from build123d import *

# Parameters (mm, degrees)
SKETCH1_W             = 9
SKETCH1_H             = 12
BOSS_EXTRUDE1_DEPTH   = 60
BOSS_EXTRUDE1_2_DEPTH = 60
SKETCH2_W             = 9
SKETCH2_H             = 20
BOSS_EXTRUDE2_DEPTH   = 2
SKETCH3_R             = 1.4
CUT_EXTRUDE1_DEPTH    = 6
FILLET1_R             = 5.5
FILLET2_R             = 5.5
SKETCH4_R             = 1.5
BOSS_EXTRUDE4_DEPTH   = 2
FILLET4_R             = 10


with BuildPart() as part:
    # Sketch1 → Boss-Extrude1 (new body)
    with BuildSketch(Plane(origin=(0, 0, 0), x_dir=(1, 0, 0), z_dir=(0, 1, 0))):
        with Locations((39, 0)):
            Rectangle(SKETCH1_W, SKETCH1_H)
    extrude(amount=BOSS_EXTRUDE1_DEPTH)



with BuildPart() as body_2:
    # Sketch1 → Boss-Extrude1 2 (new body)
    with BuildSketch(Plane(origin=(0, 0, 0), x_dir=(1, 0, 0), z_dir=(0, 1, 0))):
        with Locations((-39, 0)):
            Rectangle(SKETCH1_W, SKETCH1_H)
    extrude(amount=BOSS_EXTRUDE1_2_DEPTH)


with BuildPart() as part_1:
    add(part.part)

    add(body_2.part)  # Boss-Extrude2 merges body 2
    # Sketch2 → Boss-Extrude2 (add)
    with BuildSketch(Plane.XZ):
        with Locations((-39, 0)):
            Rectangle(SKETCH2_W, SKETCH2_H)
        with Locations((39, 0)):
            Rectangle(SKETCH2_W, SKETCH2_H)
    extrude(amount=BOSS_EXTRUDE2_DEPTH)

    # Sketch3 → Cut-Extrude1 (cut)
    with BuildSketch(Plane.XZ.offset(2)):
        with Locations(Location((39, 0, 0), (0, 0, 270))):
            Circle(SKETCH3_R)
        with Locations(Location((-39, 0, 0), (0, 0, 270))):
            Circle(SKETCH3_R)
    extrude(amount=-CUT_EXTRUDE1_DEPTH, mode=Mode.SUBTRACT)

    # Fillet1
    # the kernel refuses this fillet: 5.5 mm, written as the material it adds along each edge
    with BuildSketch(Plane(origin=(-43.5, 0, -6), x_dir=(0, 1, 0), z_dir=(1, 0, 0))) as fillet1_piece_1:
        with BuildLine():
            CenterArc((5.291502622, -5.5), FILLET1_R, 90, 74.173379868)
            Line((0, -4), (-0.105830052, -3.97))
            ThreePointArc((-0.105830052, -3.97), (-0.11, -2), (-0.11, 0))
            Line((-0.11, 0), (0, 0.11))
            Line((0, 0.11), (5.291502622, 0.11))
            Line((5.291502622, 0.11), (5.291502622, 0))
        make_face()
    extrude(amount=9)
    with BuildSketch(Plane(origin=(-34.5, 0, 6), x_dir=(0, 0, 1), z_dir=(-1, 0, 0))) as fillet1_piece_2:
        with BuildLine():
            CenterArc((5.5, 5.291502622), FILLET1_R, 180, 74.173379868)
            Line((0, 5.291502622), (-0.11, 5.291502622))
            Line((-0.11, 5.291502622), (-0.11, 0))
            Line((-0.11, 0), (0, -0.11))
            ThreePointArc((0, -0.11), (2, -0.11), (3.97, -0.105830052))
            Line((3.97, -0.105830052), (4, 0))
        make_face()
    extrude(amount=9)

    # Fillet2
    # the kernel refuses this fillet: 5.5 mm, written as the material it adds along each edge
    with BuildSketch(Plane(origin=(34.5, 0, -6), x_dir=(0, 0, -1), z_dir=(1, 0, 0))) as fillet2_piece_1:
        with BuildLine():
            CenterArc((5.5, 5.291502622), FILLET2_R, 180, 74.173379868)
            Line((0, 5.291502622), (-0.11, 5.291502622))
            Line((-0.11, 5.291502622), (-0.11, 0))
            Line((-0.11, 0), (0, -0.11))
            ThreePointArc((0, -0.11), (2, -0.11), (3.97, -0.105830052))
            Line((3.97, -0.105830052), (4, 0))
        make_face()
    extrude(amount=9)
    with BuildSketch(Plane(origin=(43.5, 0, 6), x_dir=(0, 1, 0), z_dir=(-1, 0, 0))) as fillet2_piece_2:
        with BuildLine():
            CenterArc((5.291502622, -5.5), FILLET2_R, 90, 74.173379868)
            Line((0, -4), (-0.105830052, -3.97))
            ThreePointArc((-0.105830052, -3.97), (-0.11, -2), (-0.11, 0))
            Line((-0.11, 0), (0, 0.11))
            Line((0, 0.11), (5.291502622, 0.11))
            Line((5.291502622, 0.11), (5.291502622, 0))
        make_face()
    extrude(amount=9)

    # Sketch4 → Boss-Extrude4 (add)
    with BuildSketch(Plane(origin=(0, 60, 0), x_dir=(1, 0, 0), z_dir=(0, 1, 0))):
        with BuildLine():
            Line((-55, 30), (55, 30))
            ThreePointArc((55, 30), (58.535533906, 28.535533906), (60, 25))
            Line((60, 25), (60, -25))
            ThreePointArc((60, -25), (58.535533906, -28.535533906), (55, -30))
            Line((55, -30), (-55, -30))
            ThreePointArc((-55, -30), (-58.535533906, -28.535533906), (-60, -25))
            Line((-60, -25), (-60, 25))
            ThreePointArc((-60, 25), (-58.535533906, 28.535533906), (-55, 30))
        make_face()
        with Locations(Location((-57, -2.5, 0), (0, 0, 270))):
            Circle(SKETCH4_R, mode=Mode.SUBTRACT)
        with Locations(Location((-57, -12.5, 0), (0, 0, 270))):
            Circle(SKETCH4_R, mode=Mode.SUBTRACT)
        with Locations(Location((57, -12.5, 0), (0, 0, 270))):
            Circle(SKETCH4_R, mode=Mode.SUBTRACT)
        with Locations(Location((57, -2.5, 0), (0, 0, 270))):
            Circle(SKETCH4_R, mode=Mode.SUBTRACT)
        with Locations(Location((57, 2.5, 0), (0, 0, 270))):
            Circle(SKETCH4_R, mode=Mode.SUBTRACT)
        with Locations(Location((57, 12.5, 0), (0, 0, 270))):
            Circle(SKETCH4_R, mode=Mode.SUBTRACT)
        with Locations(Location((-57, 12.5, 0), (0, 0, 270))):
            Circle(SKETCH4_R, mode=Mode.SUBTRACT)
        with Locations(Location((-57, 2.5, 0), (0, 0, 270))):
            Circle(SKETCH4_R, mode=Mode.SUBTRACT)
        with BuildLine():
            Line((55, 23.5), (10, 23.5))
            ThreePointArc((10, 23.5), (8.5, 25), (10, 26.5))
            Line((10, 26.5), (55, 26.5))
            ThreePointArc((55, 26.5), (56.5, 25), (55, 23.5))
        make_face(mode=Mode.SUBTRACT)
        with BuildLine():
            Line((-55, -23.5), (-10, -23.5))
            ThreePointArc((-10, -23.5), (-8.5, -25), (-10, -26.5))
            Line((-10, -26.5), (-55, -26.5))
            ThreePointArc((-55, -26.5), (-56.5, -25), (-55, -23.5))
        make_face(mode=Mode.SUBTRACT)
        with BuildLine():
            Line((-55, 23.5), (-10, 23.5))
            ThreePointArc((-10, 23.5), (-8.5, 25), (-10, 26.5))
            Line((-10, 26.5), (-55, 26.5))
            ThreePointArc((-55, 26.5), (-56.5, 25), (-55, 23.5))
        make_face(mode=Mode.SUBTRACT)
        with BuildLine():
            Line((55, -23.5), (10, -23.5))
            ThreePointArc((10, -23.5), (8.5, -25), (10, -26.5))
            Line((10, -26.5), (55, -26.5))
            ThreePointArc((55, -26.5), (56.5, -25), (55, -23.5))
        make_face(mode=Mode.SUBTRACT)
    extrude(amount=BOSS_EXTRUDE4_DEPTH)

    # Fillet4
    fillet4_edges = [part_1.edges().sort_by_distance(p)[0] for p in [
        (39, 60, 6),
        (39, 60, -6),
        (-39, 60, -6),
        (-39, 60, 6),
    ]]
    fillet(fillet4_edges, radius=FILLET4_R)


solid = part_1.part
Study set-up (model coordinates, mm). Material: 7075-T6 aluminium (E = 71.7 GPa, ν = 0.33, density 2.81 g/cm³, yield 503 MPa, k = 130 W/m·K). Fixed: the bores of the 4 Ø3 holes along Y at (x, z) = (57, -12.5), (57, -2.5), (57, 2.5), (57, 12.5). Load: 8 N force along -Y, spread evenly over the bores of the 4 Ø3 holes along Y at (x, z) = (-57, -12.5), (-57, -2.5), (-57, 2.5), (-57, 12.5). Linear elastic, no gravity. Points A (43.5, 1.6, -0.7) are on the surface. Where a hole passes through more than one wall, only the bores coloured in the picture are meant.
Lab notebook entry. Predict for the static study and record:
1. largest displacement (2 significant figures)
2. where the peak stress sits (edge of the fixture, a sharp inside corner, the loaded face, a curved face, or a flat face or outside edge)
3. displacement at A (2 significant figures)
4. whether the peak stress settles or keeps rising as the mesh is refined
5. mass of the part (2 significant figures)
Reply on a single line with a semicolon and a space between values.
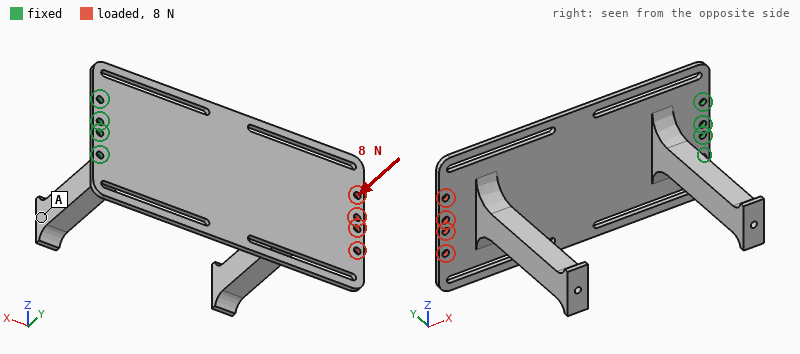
1.5 mm; edge of the fixture; 0.31 mm; keeps rising; 78 g
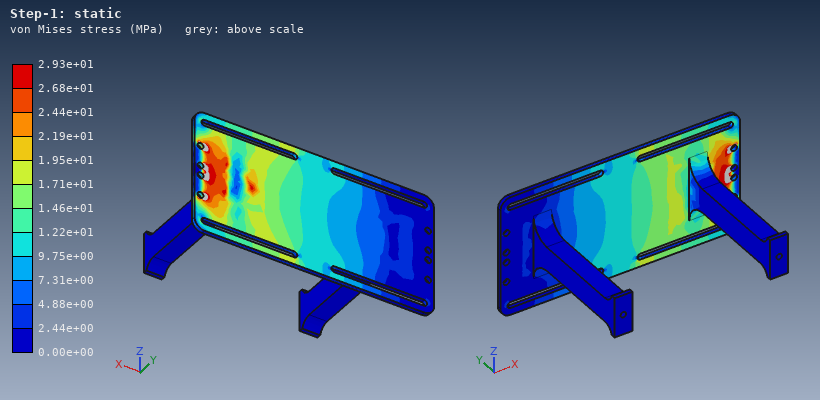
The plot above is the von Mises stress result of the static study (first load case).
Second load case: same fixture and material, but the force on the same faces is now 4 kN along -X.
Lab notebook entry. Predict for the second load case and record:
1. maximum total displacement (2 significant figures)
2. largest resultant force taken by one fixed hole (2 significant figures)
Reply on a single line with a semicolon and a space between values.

0.20 mm; 1.3 kN
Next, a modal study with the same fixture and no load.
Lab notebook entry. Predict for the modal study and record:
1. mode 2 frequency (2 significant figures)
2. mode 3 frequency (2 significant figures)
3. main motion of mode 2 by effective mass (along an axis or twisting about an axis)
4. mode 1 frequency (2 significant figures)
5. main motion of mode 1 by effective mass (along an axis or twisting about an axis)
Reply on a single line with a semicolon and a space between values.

210 Hz; 300 Hz; along Z; 76 Hz; along Y
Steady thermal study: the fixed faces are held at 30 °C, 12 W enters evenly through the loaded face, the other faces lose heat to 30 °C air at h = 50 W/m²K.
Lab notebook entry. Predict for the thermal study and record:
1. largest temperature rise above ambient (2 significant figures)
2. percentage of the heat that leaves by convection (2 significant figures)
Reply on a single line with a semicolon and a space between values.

41 K; 88 %
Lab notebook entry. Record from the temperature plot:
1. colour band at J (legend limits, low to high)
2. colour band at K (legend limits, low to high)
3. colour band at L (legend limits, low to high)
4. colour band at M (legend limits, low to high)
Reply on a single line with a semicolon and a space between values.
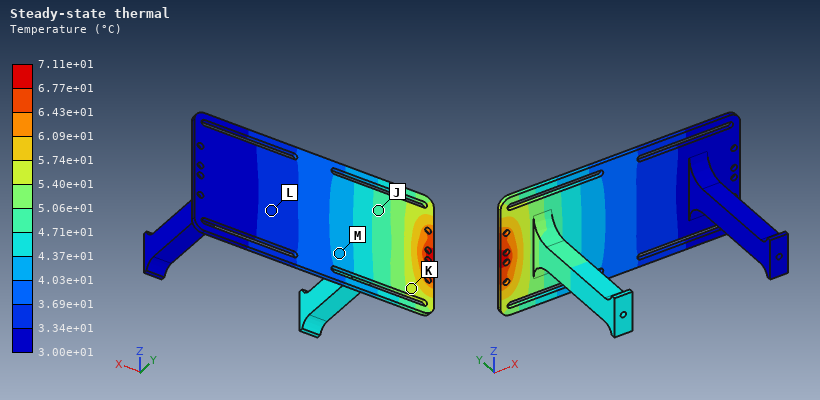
4.71e+01 to 5.06e+01 °C; 5.40e+01 to 5.74e+01 °C; 3.34e+01 to 3.69e+01 °C; 4.03e+01 to 4.37e+01 °C
